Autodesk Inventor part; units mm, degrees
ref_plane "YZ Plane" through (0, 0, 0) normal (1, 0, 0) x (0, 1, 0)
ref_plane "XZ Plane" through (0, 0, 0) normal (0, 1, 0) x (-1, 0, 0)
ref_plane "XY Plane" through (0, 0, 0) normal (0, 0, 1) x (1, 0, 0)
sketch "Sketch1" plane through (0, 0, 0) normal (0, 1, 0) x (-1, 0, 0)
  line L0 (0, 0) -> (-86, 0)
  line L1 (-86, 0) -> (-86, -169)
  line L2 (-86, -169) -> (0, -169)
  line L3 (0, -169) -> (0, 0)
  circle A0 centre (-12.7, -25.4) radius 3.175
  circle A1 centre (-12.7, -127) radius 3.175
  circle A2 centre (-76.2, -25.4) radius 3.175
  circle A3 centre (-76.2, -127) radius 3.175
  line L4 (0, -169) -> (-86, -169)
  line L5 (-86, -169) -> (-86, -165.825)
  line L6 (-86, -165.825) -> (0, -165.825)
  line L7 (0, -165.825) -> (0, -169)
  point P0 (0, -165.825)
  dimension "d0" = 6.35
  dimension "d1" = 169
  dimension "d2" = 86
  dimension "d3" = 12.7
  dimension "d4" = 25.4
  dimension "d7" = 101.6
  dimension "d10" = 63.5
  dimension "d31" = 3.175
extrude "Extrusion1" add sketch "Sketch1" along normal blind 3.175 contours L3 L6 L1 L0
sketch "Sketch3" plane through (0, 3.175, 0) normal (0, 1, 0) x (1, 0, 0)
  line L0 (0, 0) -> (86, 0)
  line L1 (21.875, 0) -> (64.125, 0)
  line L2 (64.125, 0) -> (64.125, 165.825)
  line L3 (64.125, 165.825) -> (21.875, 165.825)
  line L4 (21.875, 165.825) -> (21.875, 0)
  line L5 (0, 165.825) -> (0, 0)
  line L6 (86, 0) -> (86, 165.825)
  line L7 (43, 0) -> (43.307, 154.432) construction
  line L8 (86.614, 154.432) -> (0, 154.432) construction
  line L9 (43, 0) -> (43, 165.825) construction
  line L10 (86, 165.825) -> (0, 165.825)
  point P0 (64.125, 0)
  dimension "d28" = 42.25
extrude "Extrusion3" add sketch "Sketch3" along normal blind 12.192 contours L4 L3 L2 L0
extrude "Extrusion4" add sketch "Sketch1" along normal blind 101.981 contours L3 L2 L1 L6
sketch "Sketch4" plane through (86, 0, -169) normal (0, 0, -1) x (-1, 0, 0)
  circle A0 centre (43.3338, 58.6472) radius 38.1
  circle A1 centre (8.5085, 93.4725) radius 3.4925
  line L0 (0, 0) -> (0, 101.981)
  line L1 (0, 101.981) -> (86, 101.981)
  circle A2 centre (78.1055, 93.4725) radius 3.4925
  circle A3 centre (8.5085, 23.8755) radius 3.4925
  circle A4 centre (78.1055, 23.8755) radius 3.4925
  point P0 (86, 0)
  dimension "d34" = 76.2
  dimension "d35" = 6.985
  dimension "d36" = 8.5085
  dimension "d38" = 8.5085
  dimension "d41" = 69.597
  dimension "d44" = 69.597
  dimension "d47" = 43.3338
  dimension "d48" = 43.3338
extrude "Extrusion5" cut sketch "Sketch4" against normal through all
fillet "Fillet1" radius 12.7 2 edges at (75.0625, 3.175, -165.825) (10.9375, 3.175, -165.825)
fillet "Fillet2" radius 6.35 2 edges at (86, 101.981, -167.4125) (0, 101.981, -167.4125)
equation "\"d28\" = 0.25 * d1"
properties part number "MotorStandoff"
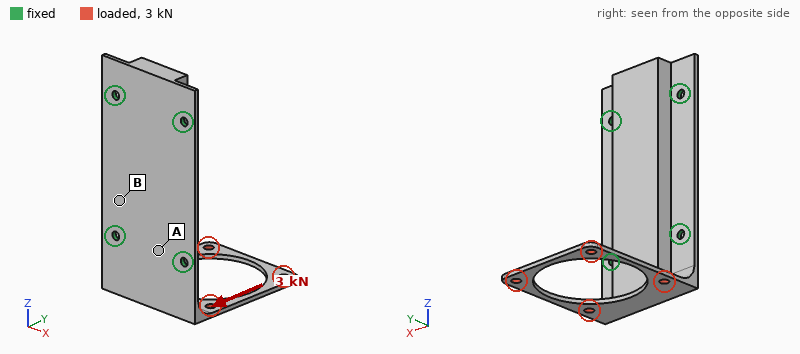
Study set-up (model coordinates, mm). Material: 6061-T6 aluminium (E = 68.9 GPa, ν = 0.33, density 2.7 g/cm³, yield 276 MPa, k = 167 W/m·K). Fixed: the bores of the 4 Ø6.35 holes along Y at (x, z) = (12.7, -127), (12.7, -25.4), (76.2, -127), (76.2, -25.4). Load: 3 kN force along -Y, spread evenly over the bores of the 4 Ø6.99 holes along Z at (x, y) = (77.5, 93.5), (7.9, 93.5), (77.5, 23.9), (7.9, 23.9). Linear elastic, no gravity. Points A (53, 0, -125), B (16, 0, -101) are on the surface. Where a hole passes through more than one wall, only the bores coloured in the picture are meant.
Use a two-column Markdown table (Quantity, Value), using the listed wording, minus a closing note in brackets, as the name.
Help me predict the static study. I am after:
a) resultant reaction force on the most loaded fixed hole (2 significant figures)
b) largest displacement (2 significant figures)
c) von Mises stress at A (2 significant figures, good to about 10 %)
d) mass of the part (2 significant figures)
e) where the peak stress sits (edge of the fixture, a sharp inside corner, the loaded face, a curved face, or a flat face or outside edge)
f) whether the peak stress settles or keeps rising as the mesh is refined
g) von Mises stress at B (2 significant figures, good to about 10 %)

| Quantity | Value |
|---|---|
| resultant reaction force on the most loaded fixed hole | 3.5 kN |
| largest displacement | 0.83 mm |
| von Mises stress at A | 41 MPa |
| mass of the part | 390 g |
| where the peak stress sits | edge of the fixture |
| whether the peak stress settles or keeps rising as the mesh is refined | keeps rising |
| von Mises stress at B | 18 MPa |
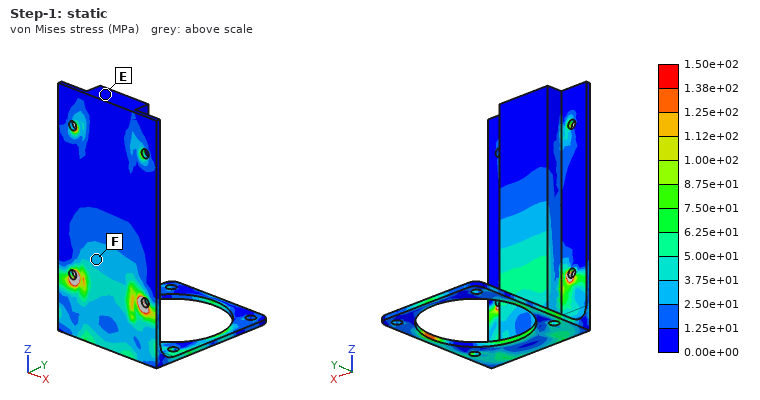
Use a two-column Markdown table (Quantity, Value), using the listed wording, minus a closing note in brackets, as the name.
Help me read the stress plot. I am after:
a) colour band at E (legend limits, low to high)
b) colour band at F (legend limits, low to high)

| Quantity | Value |
|---|---|
| colour band at E | 0.00e+00 to 1.25e+01 MPa |
| colour band at F | 2.50e+01 to 3.75e+01 MPa |
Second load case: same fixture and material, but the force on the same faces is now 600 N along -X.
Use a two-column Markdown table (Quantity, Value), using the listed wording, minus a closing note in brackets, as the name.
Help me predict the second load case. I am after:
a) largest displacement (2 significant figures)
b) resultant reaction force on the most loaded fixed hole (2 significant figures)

| Quantity | Value |
|---|---|
| largest displacement | 0.48 mm |
| resultant reaction force on the most loaded fixed hole | 750 N |
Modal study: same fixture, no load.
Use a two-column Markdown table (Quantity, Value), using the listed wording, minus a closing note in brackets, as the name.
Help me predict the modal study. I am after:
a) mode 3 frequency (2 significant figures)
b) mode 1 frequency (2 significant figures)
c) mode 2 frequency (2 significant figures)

| Quantity | Value |
|---|---|
| mode 3 frequency | 1300 Hz |
| mode 1 frequency | 230 Hz |
| mode 2 frequency | 560 Hz |
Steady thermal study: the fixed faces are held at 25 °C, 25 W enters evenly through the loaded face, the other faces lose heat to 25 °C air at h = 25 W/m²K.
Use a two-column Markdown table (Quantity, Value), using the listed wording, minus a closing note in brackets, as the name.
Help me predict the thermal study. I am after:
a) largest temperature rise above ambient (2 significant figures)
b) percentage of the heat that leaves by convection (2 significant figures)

| Quantity | Value |
|---|---|
| largest temperature rise above ambient | 76 K |
| percentage of the heat that leaves by convection | 42 % |
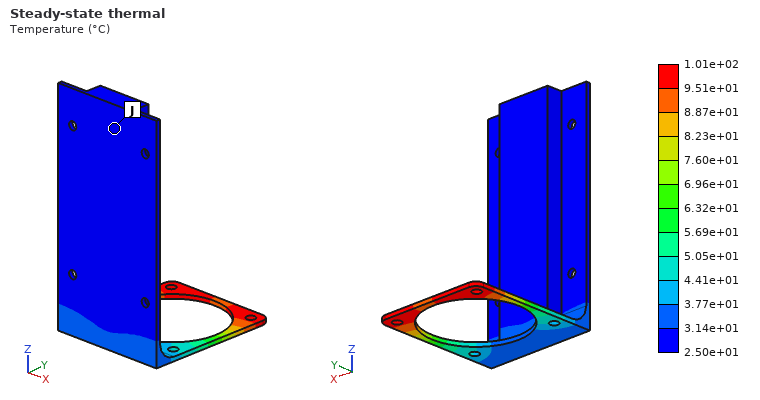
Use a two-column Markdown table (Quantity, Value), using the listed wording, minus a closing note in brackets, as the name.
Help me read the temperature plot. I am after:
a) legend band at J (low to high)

| Quantity | Value |
|---|---|
| legend band at J | 2.50e+01 to 3.14e+01 °C |
